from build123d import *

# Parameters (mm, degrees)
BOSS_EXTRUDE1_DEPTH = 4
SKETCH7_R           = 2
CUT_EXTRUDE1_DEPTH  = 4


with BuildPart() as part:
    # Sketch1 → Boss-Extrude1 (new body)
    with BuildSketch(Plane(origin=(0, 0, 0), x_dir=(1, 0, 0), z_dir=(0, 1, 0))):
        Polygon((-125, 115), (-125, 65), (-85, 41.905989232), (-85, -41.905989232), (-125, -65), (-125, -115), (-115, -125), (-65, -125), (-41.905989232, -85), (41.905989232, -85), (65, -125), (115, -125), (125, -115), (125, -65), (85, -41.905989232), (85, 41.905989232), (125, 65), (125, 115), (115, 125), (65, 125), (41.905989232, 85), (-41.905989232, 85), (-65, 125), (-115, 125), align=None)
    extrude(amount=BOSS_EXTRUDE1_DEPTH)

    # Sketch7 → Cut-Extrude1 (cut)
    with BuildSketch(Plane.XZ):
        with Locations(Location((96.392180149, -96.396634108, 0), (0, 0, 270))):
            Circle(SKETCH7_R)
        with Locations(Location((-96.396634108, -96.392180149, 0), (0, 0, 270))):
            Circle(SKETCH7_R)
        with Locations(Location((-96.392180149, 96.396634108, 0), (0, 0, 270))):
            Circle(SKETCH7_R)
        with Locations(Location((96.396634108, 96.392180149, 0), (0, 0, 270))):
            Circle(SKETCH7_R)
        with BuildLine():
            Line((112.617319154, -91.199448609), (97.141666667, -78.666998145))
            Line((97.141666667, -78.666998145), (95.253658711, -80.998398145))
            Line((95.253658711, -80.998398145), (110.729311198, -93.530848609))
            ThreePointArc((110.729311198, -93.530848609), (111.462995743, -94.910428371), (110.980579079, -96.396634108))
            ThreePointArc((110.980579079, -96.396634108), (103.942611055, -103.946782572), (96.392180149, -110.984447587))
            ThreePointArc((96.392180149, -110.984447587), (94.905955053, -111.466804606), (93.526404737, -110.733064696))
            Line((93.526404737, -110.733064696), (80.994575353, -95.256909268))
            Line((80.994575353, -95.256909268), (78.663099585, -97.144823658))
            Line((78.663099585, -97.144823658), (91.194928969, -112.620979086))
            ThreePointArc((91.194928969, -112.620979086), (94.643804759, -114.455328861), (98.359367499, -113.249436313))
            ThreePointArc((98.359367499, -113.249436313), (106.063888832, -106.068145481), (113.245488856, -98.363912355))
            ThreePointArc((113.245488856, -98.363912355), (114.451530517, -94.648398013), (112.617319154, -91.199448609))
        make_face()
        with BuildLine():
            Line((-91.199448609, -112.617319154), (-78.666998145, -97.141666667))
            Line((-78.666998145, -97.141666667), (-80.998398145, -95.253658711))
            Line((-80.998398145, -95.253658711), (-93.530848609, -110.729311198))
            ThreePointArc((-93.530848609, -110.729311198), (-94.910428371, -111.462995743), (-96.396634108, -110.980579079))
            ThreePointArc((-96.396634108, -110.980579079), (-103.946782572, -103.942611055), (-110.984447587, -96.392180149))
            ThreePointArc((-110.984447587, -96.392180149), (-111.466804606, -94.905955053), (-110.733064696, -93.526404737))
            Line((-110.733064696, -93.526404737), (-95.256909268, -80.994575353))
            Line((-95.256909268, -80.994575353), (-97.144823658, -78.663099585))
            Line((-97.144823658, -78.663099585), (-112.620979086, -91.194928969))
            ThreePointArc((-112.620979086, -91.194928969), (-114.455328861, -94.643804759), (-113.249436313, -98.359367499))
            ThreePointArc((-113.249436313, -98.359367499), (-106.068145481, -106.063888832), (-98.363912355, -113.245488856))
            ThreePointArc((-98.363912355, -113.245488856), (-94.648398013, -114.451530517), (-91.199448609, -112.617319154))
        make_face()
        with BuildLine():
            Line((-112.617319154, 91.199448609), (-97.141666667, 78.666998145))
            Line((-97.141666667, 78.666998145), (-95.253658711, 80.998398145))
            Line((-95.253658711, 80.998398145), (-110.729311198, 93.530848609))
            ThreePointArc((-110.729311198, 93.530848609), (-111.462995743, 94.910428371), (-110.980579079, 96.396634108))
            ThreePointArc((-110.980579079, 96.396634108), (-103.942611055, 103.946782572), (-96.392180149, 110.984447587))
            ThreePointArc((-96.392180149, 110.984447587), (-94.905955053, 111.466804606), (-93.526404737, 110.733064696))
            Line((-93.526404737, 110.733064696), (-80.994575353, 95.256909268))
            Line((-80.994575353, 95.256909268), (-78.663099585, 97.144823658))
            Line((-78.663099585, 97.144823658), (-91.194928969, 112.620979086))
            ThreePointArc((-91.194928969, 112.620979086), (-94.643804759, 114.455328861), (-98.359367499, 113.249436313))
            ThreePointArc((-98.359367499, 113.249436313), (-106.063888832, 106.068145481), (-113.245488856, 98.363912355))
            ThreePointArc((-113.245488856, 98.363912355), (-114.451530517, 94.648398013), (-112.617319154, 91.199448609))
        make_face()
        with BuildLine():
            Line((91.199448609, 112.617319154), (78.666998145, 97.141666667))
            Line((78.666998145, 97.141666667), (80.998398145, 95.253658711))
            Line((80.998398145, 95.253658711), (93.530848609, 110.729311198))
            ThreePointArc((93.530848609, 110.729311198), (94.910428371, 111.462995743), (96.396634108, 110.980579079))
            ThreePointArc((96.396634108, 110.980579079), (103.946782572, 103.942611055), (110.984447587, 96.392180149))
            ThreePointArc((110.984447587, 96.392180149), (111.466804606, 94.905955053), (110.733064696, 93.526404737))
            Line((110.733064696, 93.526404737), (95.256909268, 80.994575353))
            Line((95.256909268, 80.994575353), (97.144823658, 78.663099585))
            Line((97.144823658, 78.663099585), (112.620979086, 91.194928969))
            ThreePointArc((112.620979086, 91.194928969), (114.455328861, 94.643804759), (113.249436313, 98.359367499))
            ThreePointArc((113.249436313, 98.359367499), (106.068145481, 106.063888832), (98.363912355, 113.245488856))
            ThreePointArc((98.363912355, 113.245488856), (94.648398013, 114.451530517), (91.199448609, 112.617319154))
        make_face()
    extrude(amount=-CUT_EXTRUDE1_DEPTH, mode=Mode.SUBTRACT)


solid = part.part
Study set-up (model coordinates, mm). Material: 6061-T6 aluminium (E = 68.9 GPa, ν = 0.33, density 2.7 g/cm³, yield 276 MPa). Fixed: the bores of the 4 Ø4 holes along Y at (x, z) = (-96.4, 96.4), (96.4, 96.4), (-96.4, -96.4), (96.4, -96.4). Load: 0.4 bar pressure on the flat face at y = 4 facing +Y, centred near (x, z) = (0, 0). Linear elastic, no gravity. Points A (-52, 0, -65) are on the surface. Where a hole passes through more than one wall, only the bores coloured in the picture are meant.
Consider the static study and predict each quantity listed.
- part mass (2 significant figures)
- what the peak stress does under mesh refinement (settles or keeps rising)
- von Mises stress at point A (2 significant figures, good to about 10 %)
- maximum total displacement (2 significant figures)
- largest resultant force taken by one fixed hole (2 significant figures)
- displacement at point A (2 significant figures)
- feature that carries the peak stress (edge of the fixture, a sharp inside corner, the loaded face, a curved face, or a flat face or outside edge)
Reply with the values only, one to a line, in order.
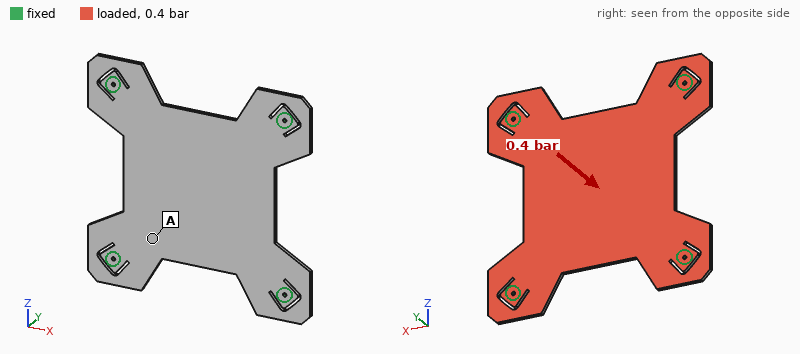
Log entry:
480 g
keeps rising
22 MPa
1.4 mm
440 N
0.74 mm
edge of the fixture
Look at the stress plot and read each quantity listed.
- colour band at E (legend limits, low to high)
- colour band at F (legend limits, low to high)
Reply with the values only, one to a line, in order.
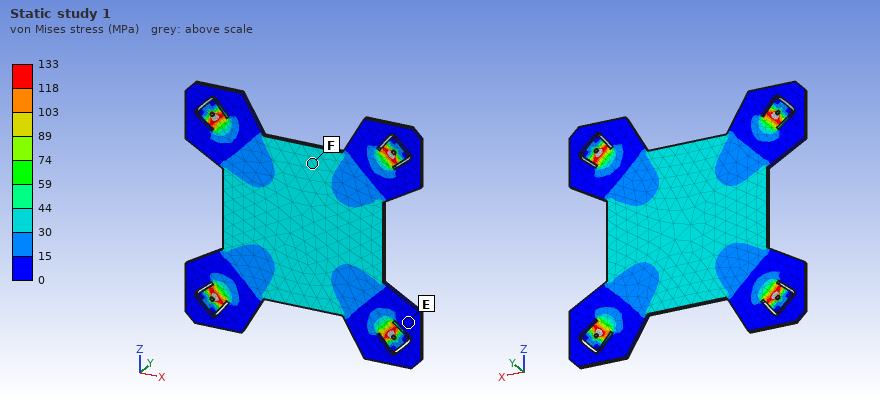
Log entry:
0 to 15 MPa
30 to 44 MPa
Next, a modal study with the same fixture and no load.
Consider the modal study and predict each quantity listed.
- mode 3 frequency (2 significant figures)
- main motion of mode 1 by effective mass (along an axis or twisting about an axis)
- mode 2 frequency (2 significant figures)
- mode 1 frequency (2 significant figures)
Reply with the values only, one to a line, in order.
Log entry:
590 Hz
along Y
590 Hz
290 Hz
